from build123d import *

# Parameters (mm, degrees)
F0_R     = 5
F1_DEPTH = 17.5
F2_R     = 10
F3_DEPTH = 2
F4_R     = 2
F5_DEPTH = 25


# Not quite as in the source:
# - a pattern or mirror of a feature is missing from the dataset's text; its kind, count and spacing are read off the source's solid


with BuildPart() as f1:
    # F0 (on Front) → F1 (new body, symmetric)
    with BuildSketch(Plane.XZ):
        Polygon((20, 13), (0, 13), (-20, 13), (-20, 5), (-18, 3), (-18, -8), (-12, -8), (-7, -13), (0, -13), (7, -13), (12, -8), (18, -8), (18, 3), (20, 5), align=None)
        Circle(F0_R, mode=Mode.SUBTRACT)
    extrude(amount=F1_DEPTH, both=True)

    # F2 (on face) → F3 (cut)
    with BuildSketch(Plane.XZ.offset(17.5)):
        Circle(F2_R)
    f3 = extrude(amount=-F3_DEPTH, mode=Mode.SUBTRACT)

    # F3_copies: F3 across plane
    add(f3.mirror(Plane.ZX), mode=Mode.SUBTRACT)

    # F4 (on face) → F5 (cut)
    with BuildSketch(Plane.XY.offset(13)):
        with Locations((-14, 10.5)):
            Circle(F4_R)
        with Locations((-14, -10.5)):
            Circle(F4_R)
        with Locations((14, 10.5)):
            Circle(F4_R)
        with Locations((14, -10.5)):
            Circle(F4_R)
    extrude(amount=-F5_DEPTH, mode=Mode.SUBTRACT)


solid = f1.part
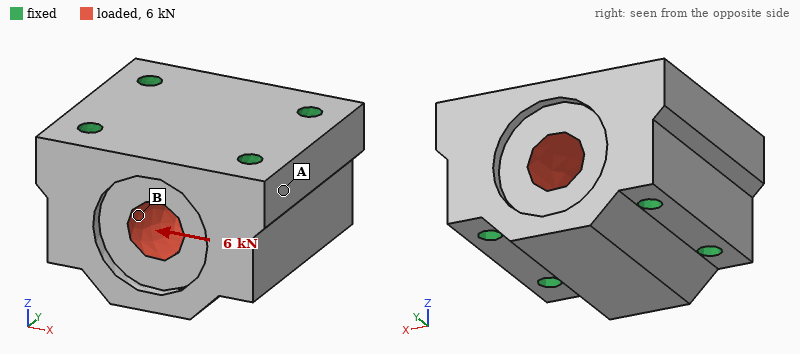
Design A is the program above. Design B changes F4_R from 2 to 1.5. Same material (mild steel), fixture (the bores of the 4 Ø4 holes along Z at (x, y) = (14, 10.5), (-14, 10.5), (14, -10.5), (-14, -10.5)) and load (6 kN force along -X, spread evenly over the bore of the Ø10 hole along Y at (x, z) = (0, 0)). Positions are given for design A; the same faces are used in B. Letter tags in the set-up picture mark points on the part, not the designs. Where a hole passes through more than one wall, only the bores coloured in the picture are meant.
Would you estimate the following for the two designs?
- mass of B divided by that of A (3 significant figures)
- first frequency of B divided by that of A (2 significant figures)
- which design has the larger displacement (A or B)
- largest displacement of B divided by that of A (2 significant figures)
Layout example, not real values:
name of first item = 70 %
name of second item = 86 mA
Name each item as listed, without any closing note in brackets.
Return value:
mass of B divided by that of A = 1.02
first frequency of B divided by that of A = 0.94
which design has the larger displacement = B
largest displacement of B divided by that of A = 1.1
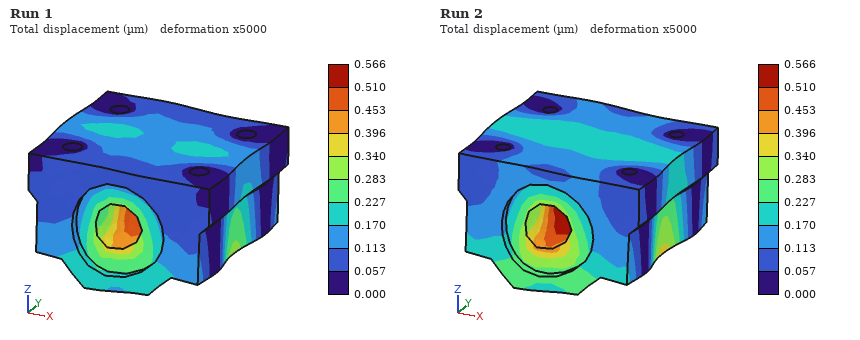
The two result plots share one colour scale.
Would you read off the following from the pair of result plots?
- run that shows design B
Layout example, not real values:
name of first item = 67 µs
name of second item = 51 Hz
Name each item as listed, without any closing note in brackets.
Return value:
run that shows design B = Run 2
